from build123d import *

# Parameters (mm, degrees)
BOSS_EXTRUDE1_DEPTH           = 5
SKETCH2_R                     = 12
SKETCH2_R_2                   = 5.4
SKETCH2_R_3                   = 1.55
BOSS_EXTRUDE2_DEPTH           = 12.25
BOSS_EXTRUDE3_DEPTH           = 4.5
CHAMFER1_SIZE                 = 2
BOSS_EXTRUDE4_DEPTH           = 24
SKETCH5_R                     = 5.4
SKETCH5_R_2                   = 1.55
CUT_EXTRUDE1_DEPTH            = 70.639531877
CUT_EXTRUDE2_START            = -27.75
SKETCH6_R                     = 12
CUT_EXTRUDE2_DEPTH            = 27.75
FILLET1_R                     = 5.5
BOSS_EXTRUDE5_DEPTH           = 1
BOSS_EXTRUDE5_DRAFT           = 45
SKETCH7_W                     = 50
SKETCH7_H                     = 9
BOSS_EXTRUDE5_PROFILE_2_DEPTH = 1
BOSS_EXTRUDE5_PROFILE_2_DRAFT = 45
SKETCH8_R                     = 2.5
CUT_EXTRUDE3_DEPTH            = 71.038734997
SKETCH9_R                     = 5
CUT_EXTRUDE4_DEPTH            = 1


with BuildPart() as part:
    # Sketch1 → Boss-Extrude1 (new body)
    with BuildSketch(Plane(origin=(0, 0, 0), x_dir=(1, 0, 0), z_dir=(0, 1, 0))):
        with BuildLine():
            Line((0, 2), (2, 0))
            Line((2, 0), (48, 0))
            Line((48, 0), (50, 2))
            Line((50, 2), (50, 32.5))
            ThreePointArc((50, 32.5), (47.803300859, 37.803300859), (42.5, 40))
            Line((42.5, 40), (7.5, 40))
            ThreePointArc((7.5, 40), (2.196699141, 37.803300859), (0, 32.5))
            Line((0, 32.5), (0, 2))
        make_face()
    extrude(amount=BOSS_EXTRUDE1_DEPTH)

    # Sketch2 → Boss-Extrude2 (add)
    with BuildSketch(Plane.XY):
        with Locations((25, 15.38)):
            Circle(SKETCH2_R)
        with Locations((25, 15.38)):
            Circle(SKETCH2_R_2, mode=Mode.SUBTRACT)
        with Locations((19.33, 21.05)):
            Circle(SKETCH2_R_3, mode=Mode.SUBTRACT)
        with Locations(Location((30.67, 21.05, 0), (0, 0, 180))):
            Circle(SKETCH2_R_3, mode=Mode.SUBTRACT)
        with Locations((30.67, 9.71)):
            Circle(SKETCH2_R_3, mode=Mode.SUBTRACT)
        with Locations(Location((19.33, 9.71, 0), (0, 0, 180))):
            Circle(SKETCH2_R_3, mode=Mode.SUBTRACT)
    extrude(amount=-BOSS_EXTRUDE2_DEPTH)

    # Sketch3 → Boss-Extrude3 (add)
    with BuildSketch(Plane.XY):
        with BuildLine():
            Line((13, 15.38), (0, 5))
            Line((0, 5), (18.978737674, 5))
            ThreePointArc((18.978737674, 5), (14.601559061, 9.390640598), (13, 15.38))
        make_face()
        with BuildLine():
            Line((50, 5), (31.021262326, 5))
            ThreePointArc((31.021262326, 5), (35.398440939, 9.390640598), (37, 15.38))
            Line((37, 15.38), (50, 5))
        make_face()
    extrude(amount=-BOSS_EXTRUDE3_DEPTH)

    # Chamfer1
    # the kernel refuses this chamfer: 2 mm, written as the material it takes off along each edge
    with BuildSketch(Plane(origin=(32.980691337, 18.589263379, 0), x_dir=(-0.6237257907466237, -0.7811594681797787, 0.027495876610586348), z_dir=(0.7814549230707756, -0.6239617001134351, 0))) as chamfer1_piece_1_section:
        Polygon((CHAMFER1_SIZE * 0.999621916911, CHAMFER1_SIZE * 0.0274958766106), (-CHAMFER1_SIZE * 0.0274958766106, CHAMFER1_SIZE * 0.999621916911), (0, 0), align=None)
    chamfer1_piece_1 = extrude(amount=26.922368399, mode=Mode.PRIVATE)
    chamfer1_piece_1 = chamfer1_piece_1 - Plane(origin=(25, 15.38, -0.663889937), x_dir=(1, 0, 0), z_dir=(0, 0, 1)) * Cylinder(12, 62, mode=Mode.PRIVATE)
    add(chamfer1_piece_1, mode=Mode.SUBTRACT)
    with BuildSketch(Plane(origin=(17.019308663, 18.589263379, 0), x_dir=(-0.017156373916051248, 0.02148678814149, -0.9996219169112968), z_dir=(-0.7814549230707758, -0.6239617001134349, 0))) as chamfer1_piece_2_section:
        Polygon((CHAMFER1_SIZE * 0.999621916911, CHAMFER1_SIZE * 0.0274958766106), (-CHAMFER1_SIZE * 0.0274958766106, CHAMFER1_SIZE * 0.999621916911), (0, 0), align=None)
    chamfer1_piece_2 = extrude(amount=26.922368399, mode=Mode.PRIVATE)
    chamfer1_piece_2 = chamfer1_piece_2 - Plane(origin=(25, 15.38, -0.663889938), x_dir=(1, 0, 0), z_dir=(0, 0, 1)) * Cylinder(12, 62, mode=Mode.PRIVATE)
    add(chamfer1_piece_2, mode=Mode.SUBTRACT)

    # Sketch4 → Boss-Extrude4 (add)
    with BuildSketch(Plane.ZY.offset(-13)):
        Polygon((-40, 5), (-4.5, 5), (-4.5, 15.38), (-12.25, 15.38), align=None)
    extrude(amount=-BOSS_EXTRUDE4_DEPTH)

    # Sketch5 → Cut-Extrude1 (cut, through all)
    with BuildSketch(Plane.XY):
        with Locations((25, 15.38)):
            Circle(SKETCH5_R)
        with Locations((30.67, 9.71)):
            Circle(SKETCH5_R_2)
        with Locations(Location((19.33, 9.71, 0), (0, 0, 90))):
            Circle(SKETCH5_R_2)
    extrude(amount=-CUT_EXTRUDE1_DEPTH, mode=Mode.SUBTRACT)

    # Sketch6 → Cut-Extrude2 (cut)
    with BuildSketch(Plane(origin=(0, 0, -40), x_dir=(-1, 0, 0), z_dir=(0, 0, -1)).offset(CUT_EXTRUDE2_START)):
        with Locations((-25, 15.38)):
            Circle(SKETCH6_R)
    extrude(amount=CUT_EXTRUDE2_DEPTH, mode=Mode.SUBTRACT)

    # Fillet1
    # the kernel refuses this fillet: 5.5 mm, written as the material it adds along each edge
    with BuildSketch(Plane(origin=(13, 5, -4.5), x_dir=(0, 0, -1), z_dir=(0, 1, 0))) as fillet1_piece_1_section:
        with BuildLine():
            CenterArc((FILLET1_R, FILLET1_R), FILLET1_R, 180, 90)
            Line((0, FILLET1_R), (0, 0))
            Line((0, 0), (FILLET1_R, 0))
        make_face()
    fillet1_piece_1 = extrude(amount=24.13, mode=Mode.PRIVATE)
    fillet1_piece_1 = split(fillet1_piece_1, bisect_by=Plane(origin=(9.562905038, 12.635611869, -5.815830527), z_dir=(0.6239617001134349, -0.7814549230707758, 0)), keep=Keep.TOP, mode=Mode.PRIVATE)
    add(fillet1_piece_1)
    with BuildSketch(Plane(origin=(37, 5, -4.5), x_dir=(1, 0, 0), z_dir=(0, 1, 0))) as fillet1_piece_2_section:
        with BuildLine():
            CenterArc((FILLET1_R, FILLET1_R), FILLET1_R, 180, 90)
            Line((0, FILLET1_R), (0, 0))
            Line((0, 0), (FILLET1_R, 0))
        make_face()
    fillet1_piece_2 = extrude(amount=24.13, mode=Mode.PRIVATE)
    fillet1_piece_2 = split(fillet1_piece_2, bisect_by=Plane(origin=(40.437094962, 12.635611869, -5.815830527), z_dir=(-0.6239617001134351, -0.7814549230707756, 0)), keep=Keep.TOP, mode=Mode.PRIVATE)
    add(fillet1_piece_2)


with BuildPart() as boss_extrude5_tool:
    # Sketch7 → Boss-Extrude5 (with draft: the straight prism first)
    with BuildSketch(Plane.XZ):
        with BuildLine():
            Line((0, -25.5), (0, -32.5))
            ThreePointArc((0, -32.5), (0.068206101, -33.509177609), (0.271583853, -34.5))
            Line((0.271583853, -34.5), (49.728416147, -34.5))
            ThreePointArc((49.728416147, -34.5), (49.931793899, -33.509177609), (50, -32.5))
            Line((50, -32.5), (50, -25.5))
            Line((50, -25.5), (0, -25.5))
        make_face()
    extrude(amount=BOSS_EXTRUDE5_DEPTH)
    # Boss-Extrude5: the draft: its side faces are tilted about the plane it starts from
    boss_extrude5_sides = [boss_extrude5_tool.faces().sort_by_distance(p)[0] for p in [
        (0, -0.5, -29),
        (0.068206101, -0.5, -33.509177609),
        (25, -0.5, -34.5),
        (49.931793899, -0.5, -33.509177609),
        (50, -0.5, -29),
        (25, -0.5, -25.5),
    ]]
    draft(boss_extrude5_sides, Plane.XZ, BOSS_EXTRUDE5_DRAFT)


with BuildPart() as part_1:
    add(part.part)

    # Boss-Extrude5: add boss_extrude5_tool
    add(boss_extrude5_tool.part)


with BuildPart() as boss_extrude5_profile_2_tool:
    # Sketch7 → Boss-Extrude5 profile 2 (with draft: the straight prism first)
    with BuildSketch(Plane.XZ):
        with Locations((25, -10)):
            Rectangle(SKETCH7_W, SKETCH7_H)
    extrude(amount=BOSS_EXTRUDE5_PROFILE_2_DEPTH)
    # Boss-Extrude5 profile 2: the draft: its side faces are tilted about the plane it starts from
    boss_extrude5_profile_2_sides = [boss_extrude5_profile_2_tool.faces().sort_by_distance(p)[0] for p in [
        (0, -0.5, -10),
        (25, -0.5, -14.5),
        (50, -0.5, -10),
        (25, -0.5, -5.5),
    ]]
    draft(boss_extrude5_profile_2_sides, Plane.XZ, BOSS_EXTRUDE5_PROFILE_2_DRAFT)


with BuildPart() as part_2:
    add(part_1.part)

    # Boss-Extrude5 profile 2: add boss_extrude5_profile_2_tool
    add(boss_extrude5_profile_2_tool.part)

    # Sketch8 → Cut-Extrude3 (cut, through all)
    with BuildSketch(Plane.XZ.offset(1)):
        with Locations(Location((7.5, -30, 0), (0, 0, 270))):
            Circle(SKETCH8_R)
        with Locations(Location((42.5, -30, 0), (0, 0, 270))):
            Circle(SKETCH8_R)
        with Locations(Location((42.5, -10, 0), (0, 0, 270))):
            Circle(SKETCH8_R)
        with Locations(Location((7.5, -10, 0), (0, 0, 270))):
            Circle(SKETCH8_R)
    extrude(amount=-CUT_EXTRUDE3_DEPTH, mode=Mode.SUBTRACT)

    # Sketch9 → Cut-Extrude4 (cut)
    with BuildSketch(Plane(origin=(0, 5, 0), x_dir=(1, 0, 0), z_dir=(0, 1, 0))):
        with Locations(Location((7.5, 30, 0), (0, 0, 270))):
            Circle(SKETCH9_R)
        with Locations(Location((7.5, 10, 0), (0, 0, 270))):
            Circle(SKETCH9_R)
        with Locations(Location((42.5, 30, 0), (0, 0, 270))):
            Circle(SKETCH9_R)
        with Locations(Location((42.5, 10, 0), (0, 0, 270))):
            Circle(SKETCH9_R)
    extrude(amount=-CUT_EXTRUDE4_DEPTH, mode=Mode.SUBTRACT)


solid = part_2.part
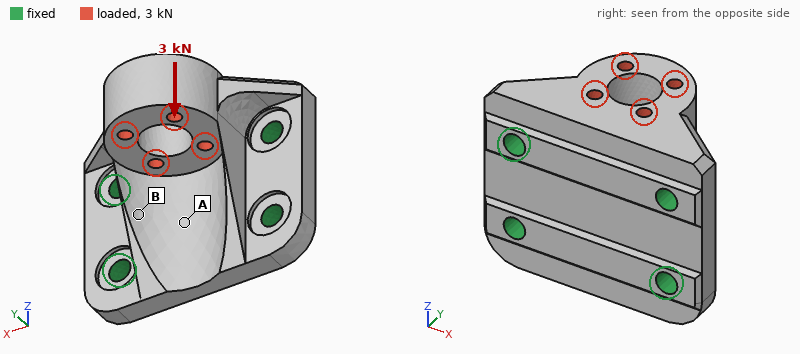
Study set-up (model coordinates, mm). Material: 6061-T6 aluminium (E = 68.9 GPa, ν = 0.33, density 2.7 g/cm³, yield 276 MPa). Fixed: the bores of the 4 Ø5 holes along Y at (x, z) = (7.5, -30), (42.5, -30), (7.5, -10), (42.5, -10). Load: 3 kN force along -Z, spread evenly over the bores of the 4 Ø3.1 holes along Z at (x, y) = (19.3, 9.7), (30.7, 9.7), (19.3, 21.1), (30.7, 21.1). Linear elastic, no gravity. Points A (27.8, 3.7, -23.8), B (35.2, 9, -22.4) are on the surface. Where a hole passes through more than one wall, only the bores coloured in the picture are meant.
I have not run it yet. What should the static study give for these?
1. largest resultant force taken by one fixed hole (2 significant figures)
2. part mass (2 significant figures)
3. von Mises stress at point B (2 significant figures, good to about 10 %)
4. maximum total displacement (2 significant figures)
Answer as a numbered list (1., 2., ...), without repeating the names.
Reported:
1. 1.3 kN
2. 41 g
3. 37 MPa
4. 85 µm
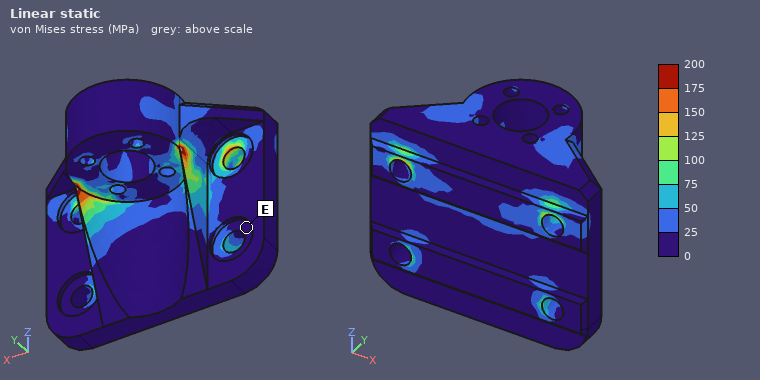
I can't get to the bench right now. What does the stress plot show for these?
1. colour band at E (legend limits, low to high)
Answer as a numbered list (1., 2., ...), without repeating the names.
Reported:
1. 0 to 25 MPa
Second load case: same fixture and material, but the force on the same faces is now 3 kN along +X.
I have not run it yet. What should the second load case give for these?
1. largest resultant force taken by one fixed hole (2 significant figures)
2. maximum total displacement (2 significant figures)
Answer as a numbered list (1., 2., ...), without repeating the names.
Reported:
1. 1.9 kN
2. 23 µm
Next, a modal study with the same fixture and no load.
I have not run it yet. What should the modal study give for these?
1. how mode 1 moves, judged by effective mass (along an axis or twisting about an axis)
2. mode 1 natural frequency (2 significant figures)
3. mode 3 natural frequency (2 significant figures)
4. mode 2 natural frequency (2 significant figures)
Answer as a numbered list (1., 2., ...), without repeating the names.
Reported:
1. along Z
2. 10 kHz
3. 19 kHz
4. 19 kHz
